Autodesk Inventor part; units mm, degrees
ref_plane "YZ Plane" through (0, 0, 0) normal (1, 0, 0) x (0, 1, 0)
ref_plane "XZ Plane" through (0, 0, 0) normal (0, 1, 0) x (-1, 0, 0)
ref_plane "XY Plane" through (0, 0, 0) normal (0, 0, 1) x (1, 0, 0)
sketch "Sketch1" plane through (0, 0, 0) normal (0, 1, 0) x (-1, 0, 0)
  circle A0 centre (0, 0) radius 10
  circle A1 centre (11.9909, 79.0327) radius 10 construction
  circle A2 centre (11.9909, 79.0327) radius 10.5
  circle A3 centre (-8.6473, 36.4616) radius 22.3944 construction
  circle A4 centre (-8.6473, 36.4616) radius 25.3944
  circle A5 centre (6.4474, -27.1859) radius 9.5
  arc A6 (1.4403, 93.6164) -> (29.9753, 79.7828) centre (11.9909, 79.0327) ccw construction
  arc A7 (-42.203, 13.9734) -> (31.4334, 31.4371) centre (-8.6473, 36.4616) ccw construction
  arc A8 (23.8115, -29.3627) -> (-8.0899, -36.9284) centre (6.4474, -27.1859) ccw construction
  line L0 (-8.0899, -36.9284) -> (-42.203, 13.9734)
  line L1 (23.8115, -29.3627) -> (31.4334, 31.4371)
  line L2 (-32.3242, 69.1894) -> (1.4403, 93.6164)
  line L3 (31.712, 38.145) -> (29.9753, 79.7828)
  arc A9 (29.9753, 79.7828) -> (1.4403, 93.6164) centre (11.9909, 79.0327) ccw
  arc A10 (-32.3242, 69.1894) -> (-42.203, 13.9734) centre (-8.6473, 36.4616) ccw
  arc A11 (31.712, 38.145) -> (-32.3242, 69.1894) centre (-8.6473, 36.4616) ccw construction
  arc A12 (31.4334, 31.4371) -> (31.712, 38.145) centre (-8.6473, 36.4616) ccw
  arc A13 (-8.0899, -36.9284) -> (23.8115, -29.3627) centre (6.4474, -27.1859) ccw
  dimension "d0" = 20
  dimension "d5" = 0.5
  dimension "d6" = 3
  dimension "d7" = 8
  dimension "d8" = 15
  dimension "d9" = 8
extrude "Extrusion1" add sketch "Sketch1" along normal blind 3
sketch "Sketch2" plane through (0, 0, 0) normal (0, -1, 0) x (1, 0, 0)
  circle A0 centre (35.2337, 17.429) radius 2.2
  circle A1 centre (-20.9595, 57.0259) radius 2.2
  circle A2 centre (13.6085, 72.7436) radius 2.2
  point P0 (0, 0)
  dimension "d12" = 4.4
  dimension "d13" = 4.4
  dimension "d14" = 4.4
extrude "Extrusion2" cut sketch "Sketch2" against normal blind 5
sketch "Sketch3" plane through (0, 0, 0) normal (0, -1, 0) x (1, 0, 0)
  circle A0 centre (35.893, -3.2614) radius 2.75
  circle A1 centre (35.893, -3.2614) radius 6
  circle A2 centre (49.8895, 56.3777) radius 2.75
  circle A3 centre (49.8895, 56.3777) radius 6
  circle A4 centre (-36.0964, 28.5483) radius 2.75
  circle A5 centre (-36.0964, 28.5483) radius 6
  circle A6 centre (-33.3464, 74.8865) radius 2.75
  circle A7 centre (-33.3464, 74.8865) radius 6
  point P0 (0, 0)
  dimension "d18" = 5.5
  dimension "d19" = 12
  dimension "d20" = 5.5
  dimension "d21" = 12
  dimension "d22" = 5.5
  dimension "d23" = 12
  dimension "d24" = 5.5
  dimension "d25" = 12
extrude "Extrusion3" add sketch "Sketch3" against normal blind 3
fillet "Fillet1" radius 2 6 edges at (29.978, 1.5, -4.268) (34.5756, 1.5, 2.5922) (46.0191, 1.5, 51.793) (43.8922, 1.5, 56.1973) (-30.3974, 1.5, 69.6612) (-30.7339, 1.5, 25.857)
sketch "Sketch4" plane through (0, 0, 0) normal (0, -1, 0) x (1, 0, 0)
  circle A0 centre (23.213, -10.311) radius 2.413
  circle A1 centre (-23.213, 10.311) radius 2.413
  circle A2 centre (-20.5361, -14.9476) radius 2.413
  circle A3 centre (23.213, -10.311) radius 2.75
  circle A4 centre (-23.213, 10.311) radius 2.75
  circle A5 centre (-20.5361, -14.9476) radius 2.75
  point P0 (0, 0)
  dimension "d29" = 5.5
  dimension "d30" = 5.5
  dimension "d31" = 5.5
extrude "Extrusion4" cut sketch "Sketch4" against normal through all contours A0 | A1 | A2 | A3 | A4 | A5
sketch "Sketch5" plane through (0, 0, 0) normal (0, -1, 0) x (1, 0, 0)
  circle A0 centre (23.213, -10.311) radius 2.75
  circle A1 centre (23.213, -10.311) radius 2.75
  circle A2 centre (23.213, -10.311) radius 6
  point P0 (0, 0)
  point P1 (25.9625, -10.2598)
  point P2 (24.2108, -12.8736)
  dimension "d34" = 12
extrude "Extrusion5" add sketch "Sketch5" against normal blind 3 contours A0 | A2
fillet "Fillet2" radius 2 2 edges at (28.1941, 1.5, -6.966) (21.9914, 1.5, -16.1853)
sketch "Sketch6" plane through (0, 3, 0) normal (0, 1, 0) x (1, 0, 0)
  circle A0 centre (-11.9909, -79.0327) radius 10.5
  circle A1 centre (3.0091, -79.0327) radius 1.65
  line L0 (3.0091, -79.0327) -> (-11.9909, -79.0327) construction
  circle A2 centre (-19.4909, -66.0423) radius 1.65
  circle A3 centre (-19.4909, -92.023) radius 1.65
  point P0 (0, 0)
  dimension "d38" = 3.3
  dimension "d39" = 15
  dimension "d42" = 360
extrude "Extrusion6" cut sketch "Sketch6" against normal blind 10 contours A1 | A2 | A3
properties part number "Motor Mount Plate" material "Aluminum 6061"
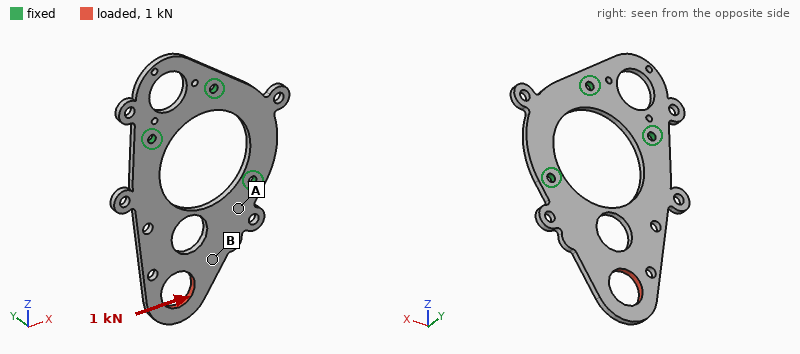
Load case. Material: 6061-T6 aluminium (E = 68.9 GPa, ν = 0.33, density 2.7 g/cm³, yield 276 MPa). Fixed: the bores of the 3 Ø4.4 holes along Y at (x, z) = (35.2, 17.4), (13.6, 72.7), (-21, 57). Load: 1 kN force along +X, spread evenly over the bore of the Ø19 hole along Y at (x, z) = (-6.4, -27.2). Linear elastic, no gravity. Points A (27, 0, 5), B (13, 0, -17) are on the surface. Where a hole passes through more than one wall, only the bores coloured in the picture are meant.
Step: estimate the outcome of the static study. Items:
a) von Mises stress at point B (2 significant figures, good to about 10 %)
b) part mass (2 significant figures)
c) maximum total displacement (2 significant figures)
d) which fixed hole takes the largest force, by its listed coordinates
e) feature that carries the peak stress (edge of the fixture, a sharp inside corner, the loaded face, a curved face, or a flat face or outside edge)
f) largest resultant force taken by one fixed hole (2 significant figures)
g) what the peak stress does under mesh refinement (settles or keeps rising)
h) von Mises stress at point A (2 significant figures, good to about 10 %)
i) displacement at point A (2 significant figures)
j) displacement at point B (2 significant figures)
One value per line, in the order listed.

10 MPa
44 g
69 µm
(35.2, 17.4)
edge of the fixture
1.2 kN
keeps rising
22 MPa
16 µm
44 µm
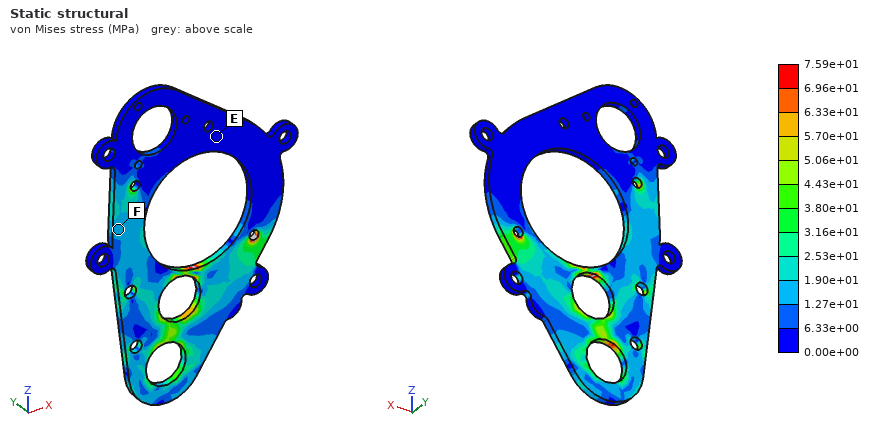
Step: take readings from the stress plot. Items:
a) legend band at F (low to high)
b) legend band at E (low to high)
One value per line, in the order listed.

1.27e+01 to 1.90e+01 MPa
0.00e+00 to 6.33e+00 MPa
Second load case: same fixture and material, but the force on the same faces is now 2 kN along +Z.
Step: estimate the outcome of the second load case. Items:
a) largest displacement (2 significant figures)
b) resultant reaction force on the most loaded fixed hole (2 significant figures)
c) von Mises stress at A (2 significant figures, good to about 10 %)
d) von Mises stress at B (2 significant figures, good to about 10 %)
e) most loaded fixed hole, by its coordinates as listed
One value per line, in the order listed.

61 µm
1.5 kN
15 MPa
15 MPa
(-21, 57)
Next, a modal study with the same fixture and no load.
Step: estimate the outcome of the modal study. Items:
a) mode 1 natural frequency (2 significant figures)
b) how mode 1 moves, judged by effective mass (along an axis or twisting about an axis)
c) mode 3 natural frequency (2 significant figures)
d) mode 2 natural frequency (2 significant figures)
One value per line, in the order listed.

450 Hz
along Y
2400 Hz
1500 Hz
